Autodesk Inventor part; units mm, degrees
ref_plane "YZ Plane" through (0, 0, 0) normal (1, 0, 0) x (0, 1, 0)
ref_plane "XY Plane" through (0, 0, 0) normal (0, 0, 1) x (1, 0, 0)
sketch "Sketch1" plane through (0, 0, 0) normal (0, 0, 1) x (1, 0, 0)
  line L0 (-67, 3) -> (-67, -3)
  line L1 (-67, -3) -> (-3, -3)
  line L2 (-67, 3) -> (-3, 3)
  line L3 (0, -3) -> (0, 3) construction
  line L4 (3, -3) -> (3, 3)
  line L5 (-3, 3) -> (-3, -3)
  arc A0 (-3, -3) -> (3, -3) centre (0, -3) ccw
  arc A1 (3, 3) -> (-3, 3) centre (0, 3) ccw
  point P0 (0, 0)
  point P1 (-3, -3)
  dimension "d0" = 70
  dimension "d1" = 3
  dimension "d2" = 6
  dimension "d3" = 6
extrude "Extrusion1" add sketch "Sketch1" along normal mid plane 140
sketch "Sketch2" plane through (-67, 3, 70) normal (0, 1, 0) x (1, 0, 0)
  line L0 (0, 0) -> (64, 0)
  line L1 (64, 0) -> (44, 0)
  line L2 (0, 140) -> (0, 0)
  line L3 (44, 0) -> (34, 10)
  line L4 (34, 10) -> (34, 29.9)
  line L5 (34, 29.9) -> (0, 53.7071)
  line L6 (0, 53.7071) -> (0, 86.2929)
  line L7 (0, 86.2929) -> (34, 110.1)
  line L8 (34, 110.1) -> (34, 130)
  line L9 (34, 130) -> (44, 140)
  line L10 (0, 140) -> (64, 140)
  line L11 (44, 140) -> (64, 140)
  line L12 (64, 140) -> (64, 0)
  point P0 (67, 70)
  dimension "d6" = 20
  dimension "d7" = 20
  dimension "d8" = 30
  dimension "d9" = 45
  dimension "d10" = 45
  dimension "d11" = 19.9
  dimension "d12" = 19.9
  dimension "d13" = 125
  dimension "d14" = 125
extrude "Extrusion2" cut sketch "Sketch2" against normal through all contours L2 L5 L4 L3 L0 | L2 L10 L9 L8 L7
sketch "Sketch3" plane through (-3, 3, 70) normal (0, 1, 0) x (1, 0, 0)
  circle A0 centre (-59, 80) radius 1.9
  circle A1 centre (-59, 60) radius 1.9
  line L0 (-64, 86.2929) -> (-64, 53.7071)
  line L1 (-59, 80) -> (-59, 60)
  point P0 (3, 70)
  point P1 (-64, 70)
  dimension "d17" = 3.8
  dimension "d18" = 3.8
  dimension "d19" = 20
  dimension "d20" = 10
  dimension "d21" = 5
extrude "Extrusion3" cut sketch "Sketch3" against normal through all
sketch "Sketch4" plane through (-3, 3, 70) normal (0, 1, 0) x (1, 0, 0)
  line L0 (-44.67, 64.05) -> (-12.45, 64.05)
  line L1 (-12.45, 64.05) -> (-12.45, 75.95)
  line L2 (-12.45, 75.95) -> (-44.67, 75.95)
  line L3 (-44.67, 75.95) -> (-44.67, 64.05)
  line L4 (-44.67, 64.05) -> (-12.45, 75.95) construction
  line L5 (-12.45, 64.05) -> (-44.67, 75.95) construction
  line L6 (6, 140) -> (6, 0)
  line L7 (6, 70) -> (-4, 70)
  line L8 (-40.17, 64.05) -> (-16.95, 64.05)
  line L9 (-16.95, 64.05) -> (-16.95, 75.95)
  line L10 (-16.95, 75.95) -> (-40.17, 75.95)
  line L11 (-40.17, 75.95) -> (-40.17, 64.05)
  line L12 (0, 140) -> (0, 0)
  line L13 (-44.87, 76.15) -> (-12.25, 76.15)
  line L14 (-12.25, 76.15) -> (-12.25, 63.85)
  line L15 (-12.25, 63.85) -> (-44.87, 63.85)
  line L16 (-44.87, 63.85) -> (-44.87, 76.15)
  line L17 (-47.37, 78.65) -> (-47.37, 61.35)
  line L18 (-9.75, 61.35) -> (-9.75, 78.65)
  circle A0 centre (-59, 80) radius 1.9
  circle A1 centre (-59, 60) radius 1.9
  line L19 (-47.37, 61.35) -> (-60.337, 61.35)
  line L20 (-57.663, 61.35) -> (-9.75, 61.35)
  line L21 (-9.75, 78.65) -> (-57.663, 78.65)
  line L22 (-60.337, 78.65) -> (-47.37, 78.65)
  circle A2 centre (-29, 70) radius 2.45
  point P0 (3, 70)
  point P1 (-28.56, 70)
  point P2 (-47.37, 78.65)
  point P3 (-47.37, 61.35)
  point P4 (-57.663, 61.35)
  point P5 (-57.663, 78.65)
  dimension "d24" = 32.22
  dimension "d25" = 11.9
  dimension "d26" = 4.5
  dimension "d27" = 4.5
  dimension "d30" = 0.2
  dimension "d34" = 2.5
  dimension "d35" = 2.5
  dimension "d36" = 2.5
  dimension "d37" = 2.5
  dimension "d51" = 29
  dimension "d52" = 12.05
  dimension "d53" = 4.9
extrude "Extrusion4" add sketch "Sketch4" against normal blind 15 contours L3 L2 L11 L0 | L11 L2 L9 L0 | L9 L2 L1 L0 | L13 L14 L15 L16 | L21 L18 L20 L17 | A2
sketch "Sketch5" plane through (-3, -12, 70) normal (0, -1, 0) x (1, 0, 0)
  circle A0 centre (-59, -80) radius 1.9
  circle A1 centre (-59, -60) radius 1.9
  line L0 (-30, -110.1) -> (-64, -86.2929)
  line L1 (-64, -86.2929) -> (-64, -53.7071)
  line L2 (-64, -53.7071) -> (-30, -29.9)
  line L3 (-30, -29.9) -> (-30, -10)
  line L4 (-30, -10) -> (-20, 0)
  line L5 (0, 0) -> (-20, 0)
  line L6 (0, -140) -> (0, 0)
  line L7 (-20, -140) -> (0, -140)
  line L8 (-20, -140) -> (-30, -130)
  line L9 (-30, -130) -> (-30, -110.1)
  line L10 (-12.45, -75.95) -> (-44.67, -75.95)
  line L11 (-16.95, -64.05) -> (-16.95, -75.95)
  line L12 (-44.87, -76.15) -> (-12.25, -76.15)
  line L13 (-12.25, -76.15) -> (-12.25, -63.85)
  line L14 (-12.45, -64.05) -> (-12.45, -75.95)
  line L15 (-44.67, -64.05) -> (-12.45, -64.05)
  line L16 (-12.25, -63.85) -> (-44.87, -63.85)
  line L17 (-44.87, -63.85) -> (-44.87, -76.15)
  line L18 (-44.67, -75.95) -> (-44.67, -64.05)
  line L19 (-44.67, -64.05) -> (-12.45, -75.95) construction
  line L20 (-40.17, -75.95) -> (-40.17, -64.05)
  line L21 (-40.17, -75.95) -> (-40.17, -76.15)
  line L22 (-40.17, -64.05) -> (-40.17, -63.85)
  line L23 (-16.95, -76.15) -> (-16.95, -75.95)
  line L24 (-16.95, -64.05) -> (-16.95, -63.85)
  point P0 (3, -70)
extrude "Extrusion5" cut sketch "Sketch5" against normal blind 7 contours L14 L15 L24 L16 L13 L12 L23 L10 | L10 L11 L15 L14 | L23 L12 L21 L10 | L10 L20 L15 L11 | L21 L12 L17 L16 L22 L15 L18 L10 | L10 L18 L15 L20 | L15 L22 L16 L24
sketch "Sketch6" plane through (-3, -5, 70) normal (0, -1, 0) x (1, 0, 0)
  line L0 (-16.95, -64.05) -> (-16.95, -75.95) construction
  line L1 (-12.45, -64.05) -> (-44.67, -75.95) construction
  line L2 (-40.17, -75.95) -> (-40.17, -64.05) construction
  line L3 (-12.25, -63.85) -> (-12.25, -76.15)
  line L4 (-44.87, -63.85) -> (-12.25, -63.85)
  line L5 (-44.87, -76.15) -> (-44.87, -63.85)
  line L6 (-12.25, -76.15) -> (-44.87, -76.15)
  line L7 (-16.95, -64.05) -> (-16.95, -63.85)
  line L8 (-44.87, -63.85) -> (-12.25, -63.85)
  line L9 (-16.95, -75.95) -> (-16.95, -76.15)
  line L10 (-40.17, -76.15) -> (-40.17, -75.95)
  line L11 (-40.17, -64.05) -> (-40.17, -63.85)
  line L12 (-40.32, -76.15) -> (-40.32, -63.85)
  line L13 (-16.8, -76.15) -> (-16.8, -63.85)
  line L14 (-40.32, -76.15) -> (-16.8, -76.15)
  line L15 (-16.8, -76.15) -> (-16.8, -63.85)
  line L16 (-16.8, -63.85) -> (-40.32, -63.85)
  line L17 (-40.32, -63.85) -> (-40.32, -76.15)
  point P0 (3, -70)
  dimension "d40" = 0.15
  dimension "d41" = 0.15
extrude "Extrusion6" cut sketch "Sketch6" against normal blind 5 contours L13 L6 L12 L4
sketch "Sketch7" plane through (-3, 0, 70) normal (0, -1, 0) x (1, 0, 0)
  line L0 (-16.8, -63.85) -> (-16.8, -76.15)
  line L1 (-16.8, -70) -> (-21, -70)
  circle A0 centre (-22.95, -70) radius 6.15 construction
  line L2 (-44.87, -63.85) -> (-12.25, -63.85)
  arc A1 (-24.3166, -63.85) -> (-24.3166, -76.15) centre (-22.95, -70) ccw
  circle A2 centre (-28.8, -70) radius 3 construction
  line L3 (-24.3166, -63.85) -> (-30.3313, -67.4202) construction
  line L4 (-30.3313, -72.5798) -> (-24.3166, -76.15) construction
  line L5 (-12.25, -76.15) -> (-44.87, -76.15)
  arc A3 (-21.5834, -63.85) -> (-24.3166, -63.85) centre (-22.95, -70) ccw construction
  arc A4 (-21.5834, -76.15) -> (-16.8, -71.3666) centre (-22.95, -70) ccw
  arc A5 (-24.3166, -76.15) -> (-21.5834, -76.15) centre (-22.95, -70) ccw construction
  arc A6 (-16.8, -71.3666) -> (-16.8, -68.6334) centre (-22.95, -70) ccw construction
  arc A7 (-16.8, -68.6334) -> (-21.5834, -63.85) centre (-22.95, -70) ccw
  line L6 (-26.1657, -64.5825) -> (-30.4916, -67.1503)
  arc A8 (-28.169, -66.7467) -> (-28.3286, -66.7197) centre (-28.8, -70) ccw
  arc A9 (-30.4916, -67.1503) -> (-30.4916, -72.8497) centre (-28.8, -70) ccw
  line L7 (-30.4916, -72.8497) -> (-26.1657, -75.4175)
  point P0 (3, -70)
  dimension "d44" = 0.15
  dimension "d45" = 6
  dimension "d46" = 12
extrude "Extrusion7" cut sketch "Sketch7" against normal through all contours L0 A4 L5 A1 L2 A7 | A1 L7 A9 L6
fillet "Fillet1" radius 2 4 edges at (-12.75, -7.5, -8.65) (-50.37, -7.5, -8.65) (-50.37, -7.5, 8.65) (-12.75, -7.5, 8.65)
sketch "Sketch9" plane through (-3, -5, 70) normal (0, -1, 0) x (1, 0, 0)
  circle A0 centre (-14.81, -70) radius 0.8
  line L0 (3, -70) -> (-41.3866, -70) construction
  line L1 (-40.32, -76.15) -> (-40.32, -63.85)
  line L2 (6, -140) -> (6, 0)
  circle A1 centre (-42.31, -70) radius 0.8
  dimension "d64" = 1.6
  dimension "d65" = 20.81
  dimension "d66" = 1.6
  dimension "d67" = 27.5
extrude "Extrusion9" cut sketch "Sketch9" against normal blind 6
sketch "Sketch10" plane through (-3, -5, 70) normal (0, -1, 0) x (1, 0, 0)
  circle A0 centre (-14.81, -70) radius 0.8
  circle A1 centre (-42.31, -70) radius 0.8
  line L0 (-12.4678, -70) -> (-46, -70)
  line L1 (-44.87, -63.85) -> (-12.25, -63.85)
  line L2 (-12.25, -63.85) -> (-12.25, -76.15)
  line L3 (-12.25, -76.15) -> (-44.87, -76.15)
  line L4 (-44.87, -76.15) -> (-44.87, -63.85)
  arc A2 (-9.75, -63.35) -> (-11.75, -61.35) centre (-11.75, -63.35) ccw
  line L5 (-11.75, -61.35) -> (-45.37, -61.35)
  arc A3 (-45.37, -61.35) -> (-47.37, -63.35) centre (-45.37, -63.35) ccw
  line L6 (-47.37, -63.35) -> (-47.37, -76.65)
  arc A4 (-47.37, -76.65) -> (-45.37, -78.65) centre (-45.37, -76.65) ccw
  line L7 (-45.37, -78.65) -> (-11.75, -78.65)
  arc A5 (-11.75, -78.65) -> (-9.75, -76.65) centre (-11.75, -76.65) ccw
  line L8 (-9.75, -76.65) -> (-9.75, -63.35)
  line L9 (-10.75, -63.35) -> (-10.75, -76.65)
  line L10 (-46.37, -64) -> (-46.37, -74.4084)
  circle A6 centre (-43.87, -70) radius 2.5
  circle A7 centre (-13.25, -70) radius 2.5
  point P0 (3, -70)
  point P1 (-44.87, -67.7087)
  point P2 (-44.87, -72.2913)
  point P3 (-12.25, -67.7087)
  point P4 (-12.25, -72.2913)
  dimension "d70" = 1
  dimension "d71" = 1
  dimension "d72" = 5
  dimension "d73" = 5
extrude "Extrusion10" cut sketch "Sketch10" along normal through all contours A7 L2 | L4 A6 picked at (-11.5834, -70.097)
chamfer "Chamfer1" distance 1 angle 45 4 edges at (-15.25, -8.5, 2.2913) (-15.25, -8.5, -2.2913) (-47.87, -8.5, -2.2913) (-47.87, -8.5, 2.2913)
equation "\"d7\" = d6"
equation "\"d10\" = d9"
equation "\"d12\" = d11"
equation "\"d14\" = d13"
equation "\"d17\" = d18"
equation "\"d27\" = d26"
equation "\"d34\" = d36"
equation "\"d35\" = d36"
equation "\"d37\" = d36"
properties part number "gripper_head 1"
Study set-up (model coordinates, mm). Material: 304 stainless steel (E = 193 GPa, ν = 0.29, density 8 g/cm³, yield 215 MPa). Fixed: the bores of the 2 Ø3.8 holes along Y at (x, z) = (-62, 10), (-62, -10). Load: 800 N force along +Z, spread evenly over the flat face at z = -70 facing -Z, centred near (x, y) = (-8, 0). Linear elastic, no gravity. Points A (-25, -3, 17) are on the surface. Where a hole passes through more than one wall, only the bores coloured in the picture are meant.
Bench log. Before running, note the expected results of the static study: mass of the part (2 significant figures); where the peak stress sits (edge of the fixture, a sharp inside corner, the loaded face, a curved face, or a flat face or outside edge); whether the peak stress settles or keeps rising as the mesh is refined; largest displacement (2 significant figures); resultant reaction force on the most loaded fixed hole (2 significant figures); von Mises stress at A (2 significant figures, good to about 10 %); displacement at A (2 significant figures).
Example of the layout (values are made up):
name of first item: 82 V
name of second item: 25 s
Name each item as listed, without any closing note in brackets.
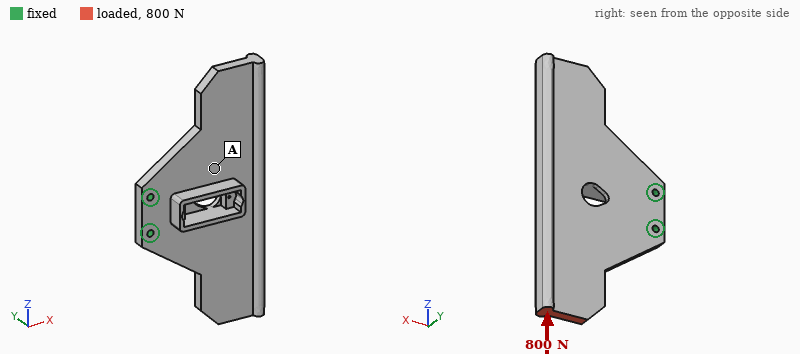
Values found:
mass of the part: 370 g
where the peak stress sits: edge of the fixture
whether the peak stress settles or keeps rising as the mesh is refined: keeps rising
largest displacement: 24 µm
resultant reaction force on the most loaded fixed hole: 1.9 kN
von Mises stress at A: 5.4 MPa
displacement at A: 9.2 µm
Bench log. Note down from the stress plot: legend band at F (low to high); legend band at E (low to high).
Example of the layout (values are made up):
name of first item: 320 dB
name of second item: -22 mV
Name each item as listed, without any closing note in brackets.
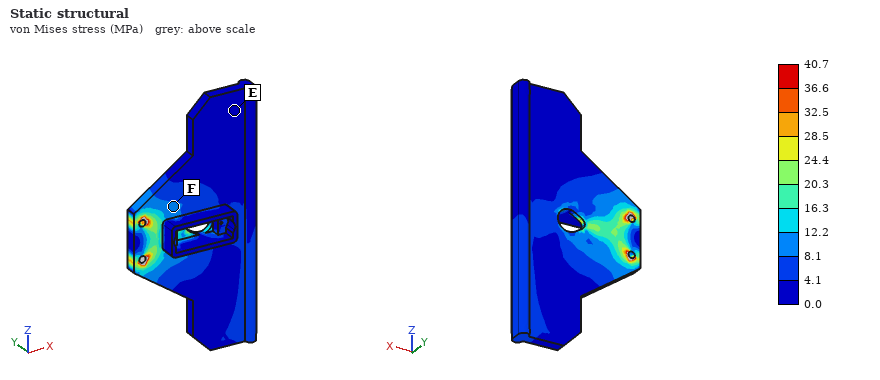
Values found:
legend band at F: 8.1 to 12.2 MPa
legend band at E: 0.0 to 4.1 MPa
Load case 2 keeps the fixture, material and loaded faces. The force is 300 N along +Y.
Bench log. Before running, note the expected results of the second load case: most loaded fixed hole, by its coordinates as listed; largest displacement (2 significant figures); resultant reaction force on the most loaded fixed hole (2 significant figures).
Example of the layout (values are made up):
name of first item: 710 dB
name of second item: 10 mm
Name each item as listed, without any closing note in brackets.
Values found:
most loaded fixed hole, by its coordinates as listed: (-62, -10)
largest displacement: 0.37 mm
resultant reaction force on the most loaded fixed hole: 850 N
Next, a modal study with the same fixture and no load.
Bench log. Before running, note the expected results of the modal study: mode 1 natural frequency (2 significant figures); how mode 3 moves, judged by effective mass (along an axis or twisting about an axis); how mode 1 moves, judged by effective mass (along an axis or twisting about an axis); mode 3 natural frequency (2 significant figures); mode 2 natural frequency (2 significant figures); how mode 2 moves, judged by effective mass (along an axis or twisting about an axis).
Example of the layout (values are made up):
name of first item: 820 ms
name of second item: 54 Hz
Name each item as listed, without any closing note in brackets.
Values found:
mode 1 natural frequency: 610 Hz
how mode 3 moves, judged by effective mass: along Z
how mode 1 moves, judged by effective mass: along Y
mode 3 natural frequency: 2000 Hz
mode 2 natural frequency: 700 Hz
how mode 2 moves, judged by effective mass: twisting about X
